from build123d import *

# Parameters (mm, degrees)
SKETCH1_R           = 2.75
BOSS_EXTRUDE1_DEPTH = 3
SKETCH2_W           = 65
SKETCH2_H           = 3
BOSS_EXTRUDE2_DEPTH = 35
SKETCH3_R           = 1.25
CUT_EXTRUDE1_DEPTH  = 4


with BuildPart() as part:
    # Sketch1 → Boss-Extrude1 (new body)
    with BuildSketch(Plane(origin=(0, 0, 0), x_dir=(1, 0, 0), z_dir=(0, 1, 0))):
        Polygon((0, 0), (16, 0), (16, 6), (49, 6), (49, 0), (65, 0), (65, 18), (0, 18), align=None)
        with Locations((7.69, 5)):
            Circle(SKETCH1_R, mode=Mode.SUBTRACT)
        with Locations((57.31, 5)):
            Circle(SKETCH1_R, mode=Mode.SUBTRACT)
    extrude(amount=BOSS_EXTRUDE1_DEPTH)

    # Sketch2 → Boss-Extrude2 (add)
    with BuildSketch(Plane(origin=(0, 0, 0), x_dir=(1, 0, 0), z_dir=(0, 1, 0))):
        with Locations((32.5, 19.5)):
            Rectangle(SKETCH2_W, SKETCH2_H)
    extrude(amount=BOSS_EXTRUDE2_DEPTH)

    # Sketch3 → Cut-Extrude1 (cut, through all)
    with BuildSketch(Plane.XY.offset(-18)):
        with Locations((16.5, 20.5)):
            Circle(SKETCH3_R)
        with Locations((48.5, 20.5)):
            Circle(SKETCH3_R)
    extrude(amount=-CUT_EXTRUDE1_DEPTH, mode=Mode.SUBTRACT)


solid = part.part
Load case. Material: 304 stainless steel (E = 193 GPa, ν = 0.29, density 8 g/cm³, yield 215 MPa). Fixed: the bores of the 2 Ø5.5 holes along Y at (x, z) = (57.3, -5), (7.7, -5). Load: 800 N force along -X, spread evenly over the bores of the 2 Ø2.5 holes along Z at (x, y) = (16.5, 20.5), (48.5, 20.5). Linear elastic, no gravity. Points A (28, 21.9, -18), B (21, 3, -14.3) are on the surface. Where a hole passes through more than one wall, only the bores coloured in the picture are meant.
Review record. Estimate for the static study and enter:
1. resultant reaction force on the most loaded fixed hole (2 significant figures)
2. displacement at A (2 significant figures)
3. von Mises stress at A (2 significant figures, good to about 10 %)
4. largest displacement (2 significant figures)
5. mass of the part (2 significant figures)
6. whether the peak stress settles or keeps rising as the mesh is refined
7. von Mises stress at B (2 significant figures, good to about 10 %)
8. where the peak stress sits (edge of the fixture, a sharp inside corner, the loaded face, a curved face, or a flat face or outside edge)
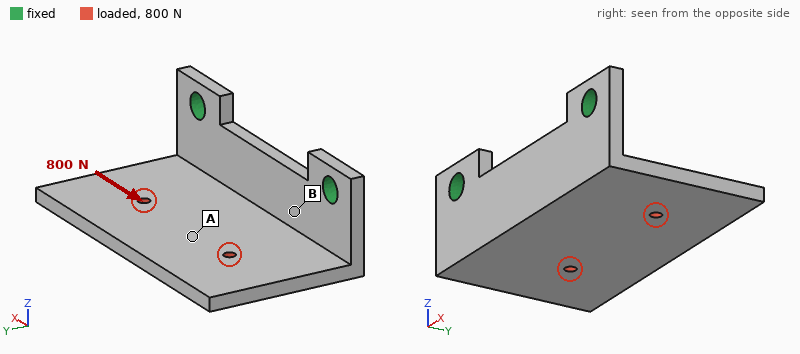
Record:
530 N
18 µm
13 MPa
46 µm
77 g
keeps rising
33 MPa
edge of the fixture
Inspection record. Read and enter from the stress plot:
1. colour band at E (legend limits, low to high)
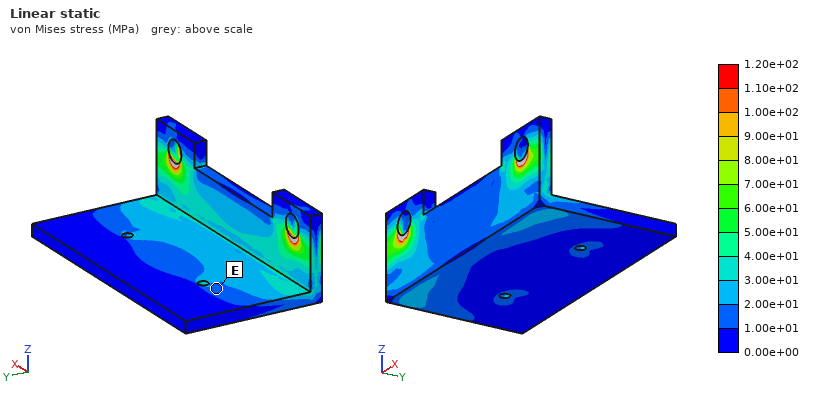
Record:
1.00e+01 to 2.00e+01 MPa
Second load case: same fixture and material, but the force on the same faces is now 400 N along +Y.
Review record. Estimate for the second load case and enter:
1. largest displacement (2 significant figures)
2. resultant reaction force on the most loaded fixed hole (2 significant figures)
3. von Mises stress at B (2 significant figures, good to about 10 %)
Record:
68 µm
200 N
12 MPa
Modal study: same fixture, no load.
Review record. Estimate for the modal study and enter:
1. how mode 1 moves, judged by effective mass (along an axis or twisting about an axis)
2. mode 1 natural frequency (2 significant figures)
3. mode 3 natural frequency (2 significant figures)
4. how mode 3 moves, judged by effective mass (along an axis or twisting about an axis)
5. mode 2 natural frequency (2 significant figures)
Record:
along Z
1200 Hz
4300 Hz
along Y
2500 Hz
